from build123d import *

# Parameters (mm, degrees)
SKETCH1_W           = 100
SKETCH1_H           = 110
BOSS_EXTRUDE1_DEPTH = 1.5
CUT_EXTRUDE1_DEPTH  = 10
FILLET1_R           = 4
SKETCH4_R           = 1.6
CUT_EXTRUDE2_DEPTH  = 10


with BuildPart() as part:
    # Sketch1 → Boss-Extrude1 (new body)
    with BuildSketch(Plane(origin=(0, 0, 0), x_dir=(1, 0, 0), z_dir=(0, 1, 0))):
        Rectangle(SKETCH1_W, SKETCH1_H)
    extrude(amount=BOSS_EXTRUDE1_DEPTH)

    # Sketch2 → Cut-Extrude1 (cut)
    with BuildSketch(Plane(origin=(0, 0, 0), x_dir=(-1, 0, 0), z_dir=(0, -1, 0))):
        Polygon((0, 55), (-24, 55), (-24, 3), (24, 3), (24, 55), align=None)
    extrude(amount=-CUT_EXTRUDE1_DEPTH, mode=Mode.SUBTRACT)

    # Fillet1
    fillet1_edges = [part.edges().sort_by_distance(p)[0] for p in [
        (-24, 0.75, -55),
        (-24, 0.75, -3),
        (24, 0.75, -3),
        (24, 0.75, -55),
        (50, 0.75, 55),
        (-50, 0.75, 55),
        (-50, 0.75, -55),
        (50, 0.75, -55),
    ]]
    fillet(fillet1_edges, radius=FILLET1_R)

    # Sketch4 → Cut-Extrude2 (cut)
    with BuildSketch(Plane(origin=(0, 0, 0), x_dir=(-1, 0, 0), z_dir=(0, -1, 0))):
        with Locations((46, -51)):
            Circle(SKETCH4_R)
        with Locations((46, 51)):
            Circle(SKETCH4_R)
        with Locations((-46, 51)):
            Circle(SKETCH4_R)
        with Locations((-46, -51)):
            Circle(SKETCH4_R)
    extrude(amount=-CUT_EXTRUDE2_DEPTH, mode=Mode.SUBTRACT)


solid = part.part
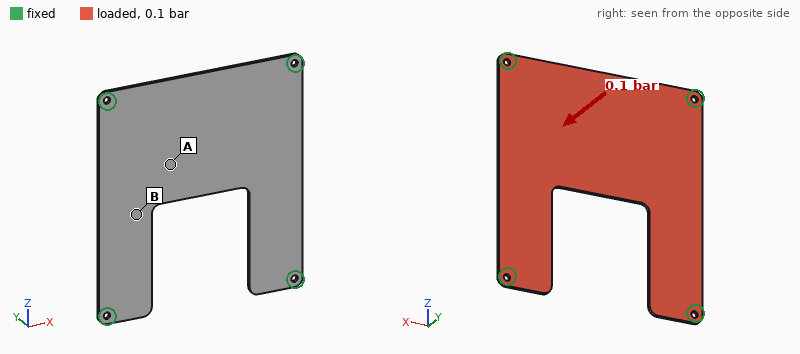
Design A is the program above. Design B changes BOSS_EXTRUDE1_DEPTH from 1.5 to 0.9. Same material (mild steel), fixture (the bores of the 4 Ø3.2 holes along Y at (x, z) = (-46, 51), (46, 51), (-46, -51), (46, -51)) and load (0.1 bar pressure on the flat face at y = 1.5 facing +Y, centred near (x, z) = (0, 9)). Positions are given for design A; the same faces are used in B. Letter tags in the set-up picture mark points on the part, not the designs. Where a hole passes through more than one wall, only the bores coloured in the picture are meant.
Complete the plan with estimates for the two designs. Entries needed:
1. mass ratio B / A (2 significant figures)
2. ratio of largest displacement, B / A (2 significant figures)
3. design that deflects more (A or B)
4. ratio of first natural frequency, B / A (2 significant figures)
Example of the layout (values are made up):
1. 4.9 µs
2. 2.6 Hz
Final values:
1. 0.60
2. 4.5
3. B
4. 0.61
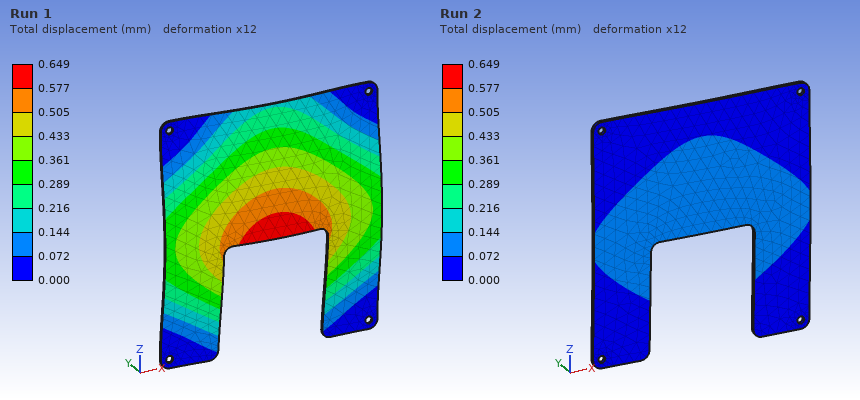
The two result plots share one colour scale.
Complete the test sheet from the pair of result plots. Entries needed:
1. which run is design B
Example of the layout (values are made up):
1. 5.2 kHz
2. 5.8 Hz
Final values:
1. Run 1
